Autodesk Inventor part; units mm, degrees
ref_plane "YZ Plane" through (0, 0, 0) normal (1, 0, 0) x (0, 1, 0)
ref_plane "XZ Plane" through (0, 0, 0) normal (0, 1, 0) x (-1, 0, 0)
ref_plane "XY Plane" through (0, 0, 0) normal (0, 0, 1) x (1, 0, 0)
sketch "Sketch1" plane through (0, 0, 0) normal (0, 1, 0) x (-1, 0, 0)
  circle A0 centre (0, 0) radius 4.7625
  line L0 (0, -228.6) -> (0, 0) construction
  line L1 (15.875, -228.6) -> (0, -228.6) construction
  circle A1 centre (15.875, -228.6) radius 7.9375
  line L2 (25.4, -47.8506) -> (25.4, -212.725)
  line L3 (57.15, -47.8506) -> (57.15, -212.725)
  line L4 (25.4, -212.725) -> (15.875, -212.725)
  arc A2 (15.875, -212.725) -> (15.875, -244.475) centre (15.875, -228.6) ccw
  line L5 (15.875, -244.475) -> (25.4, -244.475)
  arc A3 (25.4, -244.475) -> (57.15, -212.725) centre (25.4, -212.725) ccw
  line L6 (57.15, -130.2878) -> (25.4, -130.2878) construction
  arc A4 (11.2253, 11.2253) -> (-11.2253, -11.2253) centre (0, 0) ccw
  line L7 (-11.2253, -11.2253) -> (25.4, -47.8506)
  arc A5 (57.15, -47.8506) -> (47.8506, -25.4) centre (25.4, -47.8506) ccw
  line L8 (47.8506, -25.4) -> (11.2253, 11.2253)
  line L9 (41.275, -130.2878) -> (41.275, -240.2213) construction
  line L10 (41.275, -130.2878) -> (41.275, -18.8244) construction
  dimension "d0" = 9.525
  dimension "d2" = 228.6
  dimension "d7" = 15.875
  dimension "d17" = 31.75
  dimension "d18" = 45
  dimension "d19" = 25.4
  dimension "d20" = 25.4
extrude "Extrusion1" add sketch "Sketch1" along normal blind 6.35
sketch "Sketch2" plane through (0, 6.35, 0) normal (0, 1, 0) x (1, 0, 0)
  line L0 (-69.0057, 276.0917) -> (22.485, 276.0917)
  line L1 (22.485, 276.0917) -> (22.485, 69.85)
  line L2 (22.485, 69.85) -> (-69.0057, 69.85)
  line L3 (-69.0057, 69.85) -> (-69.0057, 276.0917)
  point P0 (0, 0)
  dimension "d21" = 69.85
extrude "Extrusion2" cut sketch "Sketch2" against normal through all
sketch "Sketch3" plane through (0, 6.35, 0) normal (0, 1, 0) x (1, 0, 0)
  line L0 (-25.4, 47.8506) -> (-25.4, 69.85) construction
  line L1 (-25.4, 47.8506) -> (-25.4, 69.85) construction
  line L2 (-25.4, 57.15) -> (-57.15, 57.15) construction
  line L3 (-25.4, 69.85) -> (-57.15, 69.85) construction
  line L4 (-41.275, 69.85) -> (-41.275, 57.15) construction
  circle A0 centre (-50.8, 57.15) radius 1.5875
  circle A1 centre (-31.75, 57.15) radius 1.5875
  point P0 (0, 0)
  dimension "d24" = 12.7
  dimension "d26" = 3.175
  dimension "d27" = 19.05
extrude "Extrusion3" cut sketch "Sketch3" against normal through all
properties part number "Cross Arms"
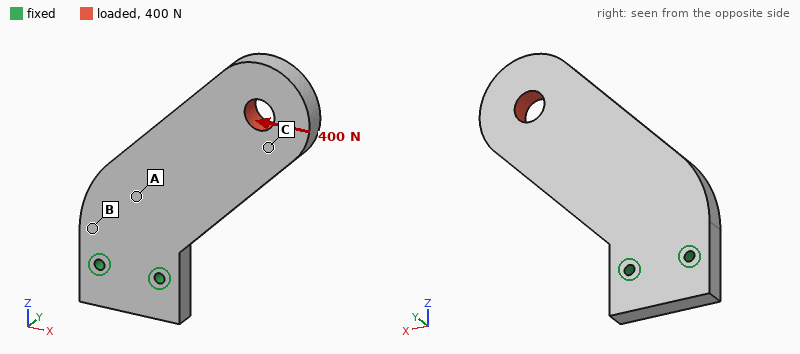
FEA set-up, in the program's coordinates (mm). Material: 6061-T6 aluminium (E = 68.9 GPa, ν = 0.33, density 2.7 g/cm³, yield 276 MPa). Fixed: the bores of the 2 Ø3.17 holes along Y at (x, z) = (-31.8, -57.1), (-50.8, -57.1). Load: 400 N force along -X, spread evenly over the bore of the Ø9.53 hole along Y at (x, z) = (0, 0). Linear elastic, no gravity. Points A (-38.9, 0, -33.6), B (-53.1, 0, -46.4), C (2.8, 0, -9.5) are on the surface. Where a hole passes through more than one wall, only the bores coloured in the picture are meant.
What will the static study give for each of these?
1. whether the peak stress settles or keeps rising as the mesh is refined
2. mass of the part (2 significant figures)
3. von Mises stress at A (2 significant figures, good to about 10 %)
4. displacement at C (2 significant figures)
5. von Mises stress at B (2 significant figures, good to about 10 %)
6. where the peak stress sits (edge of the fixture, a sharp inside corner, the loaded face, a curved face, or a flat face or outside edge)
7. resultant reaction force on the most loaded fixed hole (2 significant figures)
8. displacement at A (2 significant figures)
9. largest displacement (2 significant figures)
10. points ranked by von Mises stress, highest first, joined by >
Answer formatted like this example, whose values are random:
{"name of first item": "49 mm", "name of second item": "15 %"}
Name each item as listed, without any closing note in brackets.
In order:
{"whether the peak stress settles or keeps rising as the mesh is refined": "keeps rising", "mass of the part": "52 g", "von Mises stress at A": "7.5 MPa", "displacement at C": "37 µm", "von Mises stress at B": "12 MPa", "where the peak stress sits": "edge of the fixture", "resultant reaction force on the most loaded fixed hole": "1.1 kN", "displacement at A": "8.4 µm", "largest displacement": "54 µm", "points ranked by von Mises stress, highest first, joined by >": "B > A > C"}
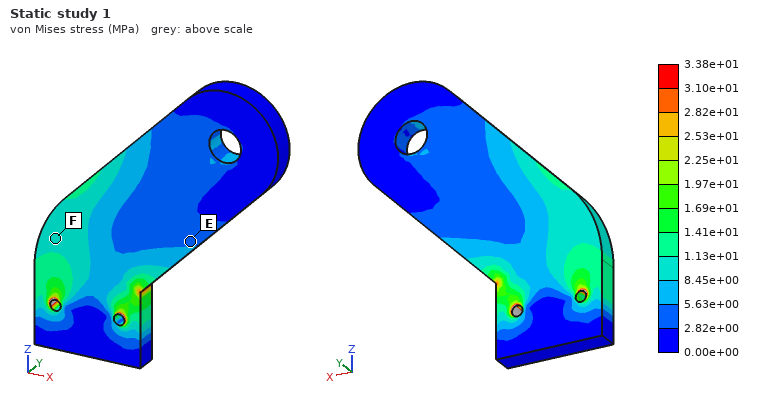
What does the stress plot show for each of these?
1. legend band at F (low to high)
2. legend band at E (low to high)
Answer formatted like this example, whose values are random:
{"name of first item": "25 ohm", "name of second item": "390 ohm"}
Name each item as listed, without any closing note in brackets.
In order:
{"legend band at F": "8.45e+00 to 1.13e+01 MPa", "legend band at E": "2.82e+00 to 5.63e+00 MPa"}
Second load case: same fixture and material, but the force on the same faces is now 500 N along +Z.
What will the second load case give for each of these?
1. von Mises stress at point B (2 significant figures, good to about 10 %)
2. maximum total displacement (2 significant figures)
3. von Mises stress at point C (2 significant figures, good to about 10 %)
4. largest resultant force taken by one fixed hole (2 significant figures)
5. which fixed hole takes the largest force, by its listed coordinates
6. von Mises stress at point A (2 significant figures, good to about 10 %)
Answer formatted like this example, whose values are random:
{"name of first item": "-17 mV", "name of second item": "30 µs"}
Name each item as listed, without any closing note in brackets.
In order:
{"von Mises stress at point B": "10 MPa", "maximum total displacement": "56 µm", "von Mises stress at point C": "5.3 MPa", "largest resultant force taken by one fixed hole": "1.3 kN", "which fixed hole takes the largest force, by its listed coordinates": "(-31.8, -57.1)", "von Mises stress at point A": "5.5 MPa"}
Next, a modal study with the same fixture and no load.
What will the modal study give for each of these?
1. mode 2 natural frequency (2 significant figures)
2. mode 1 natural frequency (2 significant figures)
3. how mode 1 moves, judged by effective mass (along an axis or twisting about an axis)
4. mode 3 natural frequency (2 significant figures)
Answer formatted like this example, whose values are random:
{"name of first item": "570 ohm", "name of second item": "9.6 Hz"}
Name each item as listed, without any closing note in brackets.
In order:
{"mode 2 natural frequency": "3200 Hz", "mode 1 natural frequency": "790 Hz", "how mode 1 moves, judged by effective mass": "along Y", "mode 3 natural frequency": "3300 Hz"}
